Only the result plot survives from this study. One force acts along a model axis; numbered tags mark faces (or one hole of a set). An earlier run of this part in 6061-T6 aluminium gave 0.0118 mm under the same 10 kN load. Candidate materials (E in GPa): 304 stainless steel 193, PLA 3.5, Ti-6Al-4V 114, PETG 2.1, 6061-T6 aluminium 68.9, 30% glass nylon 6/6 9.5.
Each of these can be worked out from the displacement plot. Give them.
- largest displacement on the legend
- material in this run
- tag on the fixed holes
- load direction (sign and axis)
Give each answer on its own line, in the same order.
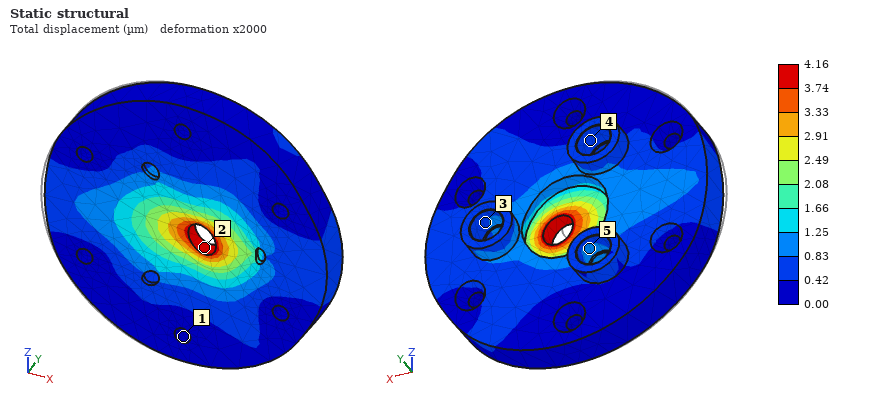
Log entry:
4.16 µm
304 stainless steel
1
+X
